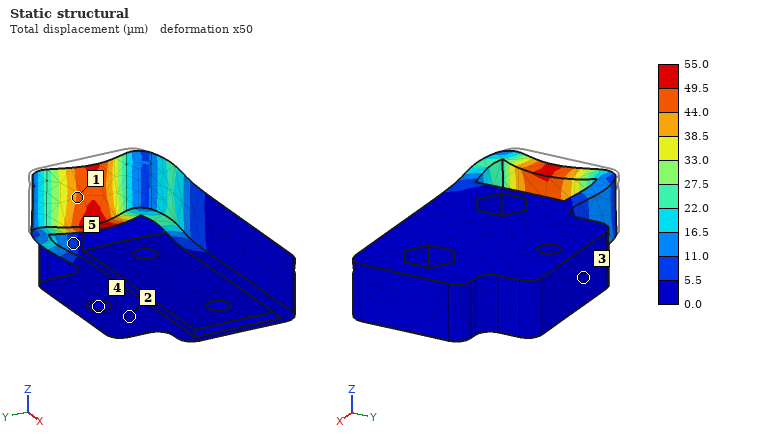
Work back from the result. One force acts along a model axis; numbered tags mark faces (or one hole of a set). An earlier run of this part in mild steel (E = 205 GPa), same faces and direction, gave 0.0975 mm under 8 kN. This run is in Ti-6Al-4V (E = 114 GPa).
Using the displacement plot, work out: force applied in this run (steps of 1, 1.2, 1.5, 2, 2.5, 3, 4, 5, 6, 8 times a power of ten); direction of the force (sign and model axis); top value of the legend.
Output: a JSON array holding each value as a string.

["2.5 kN", "+X", "55.0 µm"]
